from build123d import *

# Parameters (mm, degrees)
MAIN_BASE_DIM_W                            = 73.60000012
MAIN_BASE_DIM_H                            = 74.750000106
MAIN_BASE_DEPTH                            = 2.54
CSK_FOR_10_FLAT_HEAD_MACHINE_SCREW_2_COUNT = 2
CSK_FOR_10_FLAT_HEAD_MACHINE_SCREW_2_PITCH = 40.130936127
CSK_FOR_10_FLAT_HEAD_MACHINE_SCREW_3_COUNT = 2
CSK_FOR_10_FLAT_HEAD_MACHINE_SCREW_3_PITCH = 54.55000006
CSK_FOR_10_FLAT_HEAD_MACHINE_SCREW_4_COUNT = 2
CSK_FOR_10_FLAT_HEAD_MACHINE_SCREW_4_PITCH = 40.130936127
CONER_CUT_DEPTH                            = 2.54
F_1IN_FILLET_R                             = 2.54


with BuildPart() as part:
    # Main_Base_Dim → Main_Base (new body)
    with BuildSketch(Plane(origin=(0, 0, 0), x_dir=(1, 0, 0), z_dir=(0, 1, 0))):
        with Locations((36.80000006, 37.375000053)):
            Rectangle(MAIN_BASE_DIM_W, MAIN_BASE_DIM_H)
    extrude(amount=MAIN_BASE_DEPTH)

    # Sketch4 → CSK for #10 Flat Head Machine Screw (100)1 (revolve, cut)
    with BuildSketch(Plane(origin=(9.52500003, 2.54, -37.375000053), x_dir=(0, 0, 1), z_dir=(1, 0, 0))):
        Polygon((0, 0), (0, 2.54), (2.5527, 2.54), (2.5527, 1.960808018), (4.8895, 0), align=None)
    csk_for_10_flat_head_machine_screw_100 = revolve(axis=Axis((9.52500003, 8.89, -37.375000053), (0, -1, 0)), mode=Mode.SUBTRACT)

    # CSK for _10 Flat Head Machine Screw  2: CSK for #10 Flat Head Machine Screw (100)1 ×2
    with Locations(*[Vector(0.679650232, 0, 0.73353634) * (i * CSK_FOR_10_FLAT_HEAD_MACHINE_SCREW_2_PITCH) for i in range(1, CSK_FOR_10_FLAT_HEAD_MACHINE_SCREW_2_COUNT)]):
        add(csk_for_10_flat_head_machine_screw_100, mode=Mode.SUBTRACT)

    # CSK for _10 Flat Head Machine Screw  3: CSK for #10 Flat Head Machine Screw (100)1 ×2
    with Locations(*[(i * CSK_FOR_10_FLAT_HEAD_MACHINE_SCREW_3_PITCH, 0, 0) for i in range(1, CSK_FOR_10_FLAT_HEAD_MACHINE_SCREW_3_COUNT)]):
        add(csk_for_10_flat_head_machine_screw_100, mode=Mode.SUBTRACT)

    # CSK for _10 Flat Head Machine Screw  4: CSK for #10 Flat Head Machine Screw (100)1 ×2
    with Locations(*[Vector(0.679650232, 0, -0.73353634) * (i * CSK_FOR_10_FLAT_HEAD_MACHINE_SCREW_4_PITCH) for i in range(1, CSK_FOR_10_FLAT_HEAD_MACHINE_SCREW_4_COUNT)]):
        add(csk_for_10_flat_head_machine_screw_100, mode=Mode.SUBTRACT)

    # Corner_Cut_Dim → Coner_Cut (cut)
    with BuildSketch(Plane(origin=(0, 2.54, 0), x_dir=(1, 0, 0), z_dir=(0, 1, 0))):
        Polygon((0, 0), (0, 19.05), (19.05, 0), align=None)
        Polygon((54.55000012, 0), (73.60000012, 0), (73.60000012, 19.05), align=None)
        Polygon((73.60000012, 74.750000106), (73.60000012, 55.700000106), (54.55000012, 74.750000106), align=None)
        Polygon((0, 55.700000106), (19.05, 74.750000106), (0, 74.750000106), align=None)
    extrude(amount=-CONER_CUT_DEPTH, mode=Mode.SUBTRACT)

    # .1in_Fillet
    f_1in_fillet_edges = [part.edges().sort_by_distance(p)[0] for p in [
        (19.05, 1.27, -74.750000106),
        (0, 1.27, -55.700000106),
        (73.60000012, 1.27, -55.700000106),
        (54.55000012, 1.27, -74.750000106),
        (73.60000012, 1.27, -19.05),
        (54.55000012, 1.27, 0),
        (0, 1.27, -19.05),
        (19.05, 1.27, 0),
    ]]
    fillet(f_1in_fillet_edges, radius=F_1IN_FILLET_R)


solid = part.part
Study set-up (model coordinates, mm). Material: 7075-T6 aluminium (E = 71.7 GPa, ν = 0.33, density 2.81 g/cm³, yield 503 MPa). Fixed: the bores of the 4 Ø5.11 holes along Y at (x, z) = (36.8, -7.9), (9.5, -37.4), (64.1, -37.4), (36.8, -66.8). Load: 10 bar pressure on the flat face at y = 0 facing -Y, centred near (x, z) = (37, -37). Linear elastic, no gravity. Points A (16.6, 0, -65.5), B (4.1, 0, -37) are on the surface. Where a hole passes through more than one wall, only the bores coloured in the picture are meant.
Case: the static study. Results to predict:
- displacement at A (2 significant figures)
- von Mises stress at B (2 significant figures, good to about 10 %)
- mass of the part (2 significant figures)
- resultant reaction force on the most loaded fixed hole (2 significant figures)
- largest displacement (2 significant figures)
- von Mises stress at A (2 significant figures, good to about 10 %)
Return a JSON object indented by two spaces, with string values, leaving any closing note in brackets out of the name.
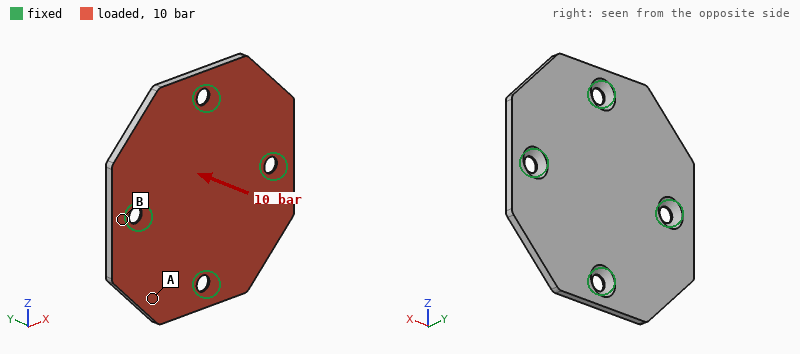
{
  "displacement at A": "0.20 mm",
  "von Mises stress at B": "140 MPa",
  "mass of the part": "33 g",
  "resultant reaction force on the most loaded fixed hole": "1.4 kN",
  "largest displacement": "0.26 mm",
  "von Mises stress at A": "63 MPa"
}
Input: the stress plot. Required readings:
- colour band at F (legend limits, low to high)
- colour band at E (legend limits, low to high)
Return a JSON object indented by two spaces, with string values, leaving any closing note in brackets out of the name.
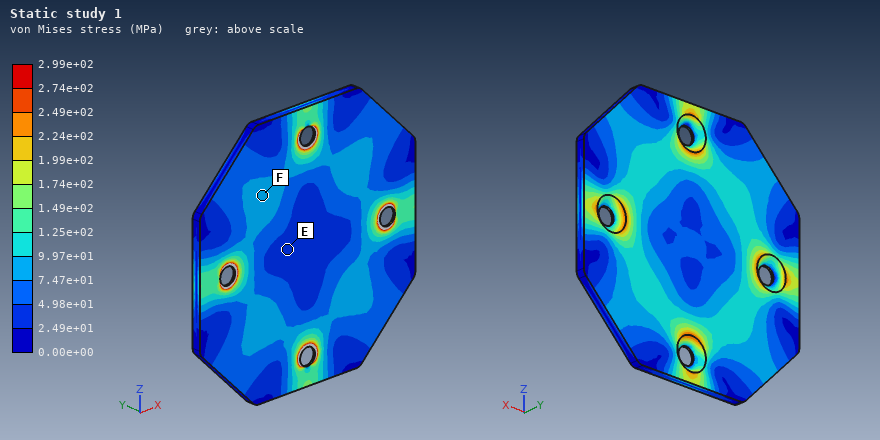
{
  "colour band at F": "7.47e+01 to 9.97e+01 MPa",
  "colour band at E": "2.49e+01 to 4.98e+01 MPa"
}
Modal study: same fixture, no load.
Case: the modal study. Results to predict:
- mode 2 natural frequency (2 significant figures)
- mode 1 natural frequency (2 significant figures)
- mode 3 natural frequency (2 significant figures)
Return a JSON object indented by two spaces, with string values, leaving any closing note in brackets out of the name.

{
  "mode 2 natural frequency": "4000 Hz",
  "mode 1 natural frequency": "3600 Hz",
  "mode 3 natural frequency": "4100 Hz"
}
